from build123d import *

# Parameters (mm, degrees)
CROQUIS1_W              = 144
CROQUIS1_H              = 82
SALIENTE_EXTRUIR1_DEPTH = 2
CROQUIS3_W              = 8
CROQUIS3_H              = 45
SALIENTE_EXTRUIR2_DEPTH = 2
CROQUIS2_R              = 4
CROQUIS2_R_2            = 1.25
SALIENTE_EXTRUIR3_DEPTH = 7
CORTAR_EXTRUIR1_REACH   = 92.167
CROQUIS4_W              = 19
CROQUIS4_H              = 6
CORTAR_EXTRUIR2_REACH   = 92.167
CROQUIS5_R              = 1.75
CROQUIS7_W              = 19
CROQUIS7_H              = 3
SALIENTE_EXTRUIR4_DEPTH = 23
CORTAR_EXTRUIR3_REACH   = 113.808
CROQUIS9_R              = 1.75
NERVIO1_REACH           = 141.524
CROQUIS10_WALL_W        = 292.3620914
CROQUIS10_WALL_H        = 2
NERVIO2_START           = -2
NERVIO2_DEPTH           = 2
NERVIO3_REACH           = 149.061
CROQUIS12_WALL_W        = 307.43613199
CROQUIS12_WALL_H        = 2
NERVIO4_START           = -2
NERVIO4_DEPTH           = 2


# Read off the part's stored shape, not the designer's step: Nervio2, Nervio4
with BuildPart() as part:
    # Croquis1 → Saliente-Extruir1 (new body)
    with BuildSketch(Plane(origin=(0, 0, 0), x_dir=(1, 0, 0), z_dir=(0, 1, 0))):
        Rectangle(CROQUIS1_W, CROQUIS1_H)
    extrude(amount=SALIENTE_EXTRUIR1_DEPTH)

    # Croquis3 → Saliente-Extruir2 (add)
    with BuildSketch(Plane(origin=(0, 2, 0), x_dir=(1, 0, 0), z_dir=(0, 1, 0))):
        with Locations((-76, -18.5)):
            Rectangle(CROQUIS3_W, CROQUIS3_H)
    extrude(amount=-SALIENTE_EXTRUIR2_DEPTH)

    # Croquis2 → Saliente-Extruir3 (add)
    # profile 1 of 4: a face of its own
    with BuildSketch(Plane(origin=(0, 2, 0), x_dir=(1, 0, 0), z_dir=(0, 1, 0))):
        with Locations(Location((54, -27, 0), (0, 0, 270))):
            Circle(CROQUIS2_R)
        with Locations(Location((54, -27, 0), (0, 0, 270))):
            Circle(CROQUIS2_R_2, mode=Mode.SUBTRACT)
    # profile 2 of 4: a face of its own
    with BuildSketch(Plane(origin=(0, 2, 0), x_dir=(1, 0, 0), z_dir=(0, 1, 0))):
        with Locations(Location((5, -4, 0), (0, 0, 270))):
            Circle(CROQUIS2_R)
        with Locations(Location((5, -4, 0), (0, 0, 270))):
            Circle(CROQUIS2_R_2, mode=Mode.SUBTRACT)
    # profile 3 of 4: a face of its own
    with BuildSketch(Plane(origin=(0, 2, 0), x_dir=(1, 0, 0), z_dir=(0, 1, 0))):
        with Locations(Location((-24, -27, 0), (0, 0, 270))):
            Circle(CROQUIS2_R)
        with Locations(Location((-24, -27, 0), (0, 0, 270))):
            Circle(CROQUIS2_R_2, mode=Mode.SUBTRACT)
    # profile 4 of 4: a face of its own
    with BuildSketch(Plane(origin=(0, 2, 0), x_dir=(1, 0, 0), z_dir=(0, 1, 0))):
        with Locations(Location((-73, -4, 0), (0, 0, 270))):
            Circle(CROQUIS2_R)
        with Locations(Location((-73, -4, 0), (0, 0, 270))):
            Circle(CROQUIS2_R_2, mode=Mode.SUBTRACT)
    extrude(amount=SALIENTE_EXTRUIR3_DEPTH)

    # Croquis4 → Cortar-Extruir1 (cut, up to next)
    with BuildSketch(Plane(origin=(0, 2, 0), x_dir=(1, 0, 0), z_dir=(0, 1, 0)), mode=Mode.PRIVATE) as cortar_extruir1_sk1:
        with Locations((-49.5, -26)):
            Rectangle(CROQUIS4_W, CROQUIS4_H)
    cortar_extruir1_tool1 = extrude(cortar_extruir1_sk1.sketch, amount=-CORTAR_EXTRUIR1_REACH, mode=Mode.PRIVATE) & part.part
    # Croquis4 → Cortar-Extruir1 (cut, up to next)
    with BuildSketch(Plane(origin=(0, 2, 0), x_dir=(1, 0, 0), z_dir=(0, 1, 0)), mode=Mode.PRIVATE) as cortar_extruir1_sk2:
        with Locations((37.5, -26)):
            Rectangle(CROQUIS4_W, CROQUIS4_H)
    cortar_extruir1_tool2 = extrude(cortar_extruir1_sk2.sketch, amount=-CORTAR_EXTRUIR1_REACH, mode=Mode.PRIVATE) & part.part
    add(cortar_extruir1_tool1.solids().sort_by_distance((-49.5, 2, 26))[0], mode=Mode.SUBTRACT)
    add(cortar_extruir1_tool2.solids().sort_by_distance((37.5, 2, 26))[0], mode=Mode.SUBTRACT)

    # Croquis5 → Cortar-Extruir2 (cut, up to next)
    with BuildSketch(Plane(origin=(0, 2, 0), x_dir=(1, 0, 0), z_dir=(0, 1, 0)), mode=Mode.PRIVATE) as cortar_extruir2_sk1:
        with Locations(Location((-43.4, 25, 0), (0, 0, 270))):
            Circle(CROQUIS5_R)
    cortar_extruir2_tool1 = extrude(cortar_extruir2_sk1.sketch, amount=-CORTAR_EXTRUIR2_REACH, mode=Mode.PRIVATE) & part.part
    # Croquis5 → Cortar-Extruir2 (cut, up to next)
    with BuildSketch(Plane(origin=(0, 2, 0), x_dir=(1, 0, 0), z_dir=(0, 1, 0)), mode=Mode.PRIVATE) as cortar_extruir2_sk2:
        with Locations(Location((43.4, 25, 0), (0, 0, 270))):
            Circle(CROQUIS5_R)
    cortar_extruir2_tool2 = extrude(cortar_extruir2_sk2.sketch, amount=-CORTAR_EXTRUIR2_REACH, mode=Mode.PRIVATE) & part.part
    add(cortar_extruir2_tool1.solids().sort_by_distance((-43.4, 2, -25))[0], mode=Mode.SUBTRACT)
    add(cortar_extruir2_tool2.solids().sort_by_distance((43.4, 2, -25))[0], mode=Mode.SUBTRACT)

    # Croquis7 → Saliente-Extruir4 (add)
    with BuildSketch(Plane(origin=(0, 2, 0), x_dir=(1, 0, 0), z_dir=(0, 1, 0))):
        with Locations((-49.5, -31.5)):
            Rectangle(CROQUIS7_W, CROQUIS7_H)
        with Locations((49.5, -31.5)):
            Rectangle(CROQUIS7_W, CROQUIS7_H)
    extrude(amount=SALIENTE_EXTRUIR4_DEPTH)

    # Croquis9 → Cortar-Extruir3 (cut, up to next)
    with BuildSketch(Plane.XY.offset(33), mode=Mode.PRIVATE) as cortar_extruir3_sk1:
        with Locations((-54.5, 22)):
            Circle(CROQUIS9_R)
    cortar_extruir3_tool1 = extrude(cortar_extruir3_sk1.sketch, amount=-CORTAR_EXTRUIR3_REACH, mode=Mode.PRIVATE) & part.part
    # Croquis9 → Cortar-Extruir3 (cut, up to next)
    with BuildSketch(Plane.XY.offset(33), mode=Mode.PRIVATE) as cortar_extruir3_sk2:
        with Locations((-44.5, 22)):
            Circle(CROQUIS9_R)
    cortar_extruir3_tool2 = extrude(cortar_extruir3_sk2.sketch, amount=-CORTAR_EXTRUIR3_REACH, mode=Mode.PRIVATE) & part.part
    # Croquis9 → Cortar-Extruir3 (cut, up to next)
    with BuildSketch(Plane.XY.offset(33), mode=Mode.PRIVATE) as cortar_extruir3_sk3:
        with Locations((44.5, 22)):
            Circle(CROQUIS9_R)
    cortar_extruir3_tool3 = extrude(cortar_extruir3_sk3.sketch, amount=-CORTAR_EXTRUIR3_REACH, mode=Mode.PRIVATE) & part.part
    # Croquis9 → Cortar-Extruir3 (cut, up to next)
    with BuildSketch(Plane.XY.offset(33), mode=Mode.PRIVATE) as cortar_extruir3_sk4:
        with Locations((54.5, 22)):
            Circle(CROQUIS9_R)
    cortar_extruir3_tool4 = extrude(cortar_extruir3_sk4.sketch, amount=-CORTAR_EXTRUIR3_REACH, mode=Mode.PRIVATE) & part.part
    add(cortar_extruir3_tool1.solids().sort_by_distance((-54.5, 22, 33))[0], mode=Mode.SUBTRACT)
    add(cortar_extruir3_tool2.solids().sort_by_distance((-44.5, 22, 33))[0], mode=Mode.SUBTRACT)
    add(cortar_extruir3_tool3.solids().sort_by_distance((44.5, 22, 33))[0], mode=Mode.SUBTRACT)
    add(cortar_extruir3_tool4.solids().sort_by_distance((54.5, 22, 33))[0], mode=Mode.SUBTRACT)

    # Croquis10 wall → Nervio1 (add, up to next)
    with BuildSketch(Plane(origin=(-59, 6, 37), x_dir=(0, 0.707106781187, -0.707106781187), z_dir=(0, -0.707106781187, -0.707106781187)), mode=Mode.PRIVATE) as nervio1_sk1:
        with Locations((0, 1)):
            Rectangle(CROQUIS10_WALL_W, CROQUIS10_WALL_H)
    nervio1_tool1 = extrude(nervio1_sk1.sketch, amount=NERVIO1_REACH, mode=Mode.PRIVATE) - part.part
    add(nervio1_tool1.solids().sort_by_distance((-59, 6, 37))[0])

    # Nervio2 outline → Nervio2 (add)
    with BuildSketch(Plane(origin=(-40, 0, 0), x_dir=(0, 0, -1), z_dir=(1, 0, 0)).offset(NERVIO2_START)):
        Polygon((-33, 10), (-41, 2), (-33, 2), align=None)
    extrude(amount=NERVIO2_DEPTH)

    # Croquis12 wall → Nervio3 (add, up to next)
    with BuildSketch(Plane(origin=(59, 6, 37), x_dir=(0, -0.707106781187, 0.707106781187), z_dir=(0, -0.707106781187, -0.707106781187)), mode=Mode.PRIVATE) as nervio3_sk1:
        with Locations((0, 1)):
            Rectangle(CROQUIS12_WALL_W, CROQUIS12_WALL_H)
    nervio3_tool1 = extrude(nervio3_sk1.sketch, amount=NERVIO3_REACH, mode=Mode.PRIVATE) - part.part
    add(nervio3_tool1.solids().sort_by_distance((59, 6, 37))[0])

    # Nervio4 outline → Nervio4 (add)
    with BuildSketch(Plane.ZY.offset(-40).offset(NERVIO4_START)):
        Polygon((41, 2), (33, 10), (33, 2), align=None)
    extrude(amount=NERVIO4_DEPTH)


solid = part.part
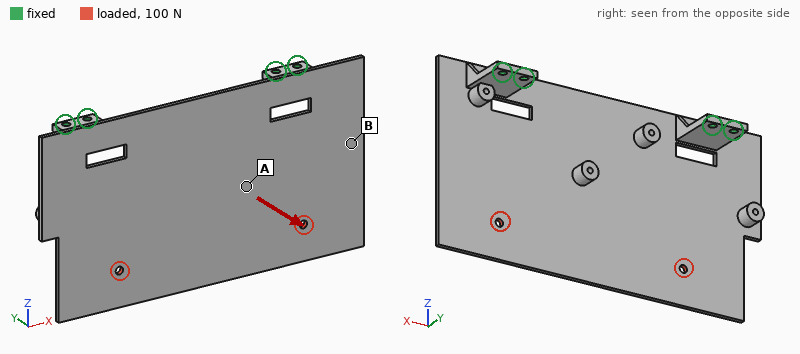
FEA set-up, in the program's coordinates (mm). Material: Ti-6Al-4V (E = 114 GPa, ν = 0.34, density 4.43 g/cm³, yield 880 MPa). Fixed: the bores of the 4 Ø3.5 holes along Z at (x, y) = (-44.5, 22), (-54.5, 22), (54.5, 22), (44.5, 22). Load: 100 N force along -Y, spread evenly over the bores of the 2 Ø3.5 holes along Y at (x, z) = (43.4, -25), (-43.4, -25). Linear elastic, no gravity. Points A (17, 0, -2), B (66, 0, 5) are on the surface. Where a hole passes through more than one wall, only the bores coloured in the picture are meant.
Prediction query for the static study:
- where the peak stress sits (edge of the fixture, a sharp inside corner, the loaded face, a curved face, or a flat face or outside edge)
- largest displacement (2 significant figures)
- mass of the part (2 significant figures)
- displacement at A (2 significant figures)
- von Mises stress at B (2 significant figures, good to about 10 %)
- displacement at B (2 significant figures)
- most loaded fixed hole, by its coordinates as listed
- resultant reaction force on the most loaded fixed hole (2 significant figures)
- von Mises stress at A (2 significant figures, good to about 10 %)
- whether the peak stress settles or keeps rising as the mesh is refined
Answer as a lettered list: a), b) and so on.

a) a sharp inside corner
b) 1.8 mm
c) 120 g
d) 0.72 mm
e) 50 MPa
f) 0.38 mm
g) (54.5, 22)
h) 49 N
i) 21 MPa
j) keeps rising
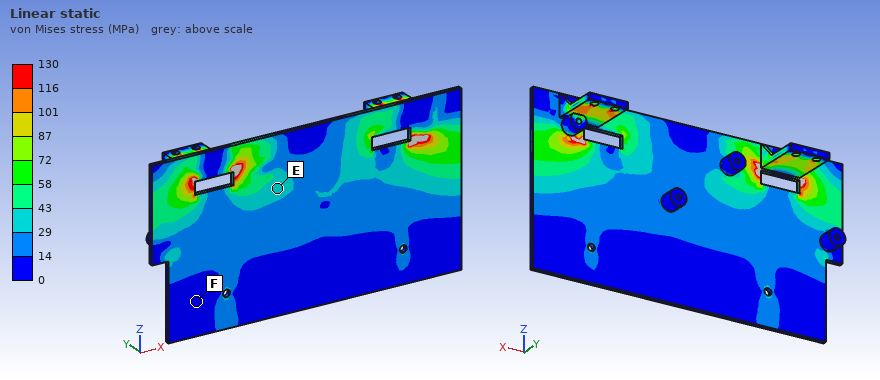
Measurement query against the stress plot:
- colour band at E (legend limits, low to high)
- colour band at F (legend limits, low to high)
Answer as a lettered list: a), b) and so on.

a) 29 to 43 MPa
b) 0 to 14 MPa
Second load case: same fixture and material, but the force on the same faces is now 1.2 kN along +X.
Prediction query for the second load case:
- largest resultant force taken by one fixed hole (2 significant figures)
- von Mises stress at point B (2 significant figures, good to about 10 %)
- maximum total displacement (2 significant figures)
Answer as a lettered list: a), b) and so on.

a) 1.2 kN
b) 38 MPa
c) 1.0 mm
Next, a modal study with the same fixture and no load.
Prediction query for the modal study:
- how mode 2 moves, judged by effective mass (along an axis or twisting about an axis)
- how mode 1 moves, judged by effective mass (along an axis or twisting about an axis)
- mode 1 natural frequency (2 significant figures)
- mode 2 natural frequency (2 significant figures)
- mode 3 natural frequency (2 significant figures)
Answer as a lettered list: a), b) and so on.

a) twisting about Z
b) along Y
c) 200 Hz
d) 410 Hz
e) 790 Hz
